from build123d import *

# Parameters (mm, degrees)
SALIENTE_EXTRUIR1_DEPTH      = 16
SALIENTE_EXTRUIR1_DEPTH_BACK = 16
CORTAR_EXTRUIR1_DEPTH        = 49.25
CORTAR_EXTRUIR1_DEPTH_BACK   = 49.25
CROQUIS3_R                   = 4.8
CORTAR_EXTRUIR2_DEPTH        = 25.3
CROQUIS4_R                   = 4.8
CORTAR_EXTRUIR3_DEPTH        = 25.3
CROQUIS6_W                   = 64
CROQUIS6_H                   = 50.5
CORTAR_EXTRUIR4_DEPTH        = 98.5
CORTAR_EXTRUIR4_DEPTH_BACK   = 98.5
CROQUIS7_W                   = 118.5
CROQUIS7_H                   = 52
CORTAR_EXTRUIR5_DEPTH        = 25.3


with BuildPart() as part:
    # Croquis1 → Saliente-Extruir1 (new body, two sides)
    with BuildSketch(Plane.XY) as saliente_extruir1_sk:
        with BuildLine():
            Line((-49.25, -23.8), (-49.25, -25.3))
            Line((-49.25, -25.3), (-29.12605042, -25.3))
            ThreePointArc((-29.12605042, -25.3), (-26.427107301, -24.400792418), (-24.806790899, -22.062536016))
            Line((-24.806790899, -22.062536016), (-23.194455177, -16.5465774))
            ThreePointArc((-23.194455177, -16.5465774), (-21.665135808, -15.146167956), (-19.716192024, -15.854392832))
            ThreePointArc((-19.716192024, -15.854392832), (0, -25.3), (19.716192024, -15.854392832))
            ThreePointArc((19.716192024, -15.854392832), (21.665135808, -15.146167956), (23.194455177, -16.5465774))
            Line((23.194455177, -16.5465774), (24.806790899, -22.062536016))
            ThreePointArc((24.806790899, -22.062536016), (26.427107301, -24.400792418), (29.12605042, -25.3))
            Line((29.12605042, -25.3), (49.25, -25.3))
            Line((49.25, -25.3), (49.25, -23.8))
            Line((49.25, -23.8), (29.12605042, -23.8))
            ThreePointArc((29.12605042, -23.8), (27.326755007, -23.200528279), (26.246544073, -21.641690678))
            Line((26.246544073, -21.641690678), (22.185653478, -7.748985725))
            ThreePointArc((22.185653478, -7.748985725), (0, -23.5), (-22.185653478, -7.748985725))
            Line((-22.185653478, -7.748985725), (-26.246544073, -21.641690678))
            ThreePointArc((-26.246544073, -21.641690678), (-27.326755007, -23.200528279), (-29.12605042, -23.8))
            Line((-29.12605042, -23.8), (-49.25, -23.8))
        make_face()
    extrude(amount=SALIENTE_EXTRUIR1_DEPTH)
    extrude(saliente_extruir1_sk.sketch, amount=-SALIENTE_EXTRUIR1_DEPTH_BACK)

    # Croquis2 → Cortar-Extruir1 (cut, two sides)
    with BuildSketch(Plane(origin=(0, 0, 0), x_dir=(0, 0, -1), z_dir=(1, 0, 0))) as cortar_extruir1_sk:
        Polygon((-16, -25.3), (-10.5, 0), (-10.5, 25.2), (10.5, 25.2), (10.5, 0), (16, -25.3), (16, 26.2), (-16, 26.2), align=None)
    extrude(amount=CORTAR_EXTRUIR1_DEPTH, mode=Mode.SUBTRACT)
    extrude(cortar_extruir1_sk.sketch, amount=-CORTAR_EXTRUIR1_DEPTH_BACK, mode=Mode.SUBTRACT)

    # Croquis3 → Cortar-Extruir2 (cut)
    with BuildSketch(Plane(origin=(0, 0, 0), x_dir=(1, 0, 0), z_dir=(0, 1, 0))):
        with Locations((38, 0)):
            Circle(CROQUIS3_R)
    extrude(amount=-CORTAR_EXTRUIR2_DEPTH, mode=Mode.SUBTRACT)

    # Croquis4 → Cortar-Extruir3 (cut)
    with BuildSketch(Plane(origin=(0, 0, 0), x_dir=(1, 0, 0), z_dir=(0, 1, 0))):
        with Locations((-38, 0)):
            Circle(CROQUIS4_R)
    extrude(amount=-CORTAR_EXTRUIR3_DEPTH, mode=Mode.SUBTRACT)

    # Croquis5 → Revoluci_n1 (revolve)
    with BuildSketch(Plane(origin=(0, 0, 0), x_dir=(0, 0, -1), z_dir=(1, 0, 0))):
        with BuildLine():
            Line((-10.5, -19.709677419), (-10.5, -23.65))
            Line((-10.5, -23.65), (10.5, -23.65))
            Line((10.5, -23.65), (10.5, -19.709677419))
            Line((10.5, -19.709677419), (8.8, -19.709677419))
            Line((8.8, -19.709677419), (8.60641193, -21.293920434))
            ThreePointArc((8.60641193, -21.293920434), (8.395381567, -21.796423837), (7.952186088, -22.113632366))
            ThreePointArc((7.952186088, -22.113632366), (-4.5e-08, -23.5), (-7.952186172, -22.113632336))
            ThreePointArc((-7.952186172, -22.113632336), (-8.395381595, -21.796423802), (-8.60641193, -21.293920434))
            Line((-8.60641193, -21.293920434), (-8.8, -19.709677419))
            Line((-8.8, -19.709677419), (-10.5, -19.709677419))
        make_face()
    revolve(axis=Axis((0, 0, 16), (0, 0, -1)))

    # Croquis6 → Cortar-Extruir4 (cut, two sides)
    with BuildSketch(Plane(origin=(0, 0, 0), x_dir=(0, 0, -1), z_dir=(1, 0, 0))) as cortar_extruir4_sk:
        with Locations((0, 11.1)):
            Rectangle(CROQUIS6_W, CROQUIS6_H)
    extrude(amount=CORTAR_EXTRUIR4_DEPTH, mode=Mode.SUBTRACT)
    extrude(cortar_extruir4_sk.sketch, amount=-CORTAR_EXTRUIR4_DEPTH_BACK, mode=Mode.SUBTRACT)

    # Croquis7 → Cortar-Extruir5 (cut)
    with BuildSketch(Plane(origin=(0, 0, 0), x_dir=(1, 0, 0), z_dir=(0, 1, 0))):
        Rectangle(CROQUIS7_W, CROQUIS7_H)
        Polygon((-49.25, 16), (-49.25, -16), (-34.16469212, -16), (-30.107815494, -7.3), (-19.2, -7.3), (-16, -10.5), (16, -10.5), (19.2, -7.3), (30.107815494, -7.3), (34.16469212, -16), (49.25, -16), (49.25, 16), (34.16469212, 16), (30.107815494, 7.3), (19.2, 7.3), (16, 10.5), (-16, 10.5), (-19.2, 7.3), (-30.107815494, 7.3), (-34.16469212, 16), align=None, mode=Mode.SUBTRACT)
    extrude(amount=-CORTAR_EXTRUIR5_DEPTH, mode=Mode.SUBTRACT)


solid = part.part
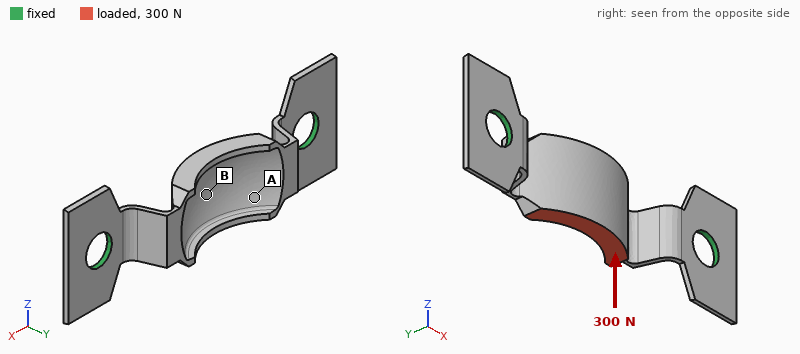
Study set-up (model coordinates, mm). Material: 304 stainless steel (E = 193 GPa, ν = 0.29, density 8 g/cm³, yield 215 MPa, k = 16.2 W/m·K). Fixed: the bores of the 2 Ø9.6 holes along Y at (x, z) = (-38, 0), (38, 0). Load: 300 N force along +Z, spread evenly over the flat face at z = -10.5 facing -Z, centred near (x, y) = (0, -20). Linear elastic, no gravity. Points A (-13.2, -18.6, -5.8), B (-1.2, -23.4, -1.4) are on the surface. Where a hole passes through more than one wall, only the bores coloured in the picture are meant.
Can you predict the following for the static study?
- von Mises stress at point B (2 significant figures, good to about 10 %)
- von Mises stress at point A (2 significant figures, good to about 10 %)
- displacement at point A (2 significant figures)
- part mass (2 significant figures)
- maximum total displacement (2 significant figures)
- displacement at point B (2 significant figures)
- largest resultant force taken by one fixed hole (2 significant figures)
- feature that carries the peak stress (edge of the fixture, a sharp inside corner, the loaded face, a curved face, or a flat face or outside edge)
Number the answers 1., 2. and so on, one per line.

1. 9.6 MPa
2. 18 MPa
3. 27 µm
4. 38 g
5. 41 µm
6. 33 µm
7. 150 N
8. a flat face or outside edge
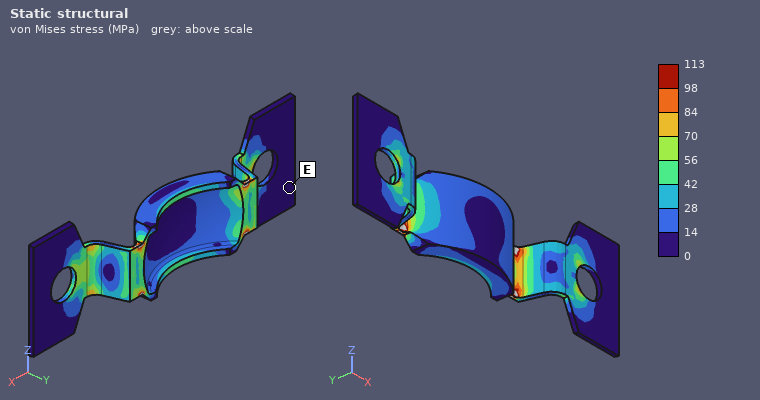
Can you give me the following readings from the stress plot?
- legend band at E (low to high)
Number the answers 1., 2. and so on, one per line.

1. 0 to 14 MPa
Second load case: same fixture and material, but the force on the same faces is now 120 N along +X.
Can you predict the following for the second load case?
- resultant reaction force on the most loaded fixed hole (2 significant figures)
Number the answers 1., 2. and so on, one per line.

1. 65 N
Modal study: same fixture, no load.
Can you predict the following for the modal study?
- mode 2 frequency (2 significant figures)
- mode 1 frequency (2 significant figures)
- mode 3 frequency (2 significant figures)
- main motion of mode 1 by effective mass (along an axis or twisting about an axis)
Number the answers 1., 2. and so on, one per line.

1. 2500 Hz
2. 1800 Hz
3. 2600 Hz
4. along X
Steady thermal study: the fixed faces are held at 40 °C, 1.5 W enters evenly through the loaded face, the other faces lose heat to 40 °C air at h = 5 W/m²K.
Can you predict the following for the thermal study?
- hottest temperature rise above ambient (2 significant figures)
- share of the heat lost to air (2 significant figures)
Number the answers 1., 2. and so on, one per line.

1. 47 K
2. 35 %
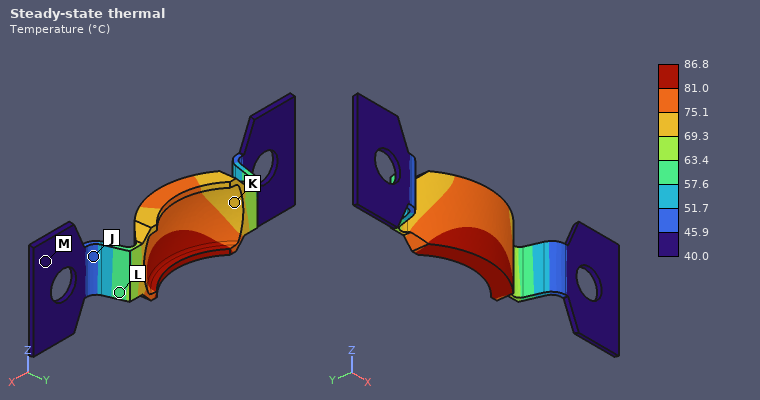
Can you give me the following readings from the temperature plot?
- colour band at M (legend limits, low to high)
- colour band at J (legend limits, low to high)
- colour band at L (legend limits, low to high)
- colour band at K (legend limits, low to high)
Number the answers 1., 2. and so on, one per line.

1. 40.0 to 45.9 °C
2. 45.9 to 51.7 °C
3. 57.6 to 63.4 °C
4. 69.3 to 75.1 °C
